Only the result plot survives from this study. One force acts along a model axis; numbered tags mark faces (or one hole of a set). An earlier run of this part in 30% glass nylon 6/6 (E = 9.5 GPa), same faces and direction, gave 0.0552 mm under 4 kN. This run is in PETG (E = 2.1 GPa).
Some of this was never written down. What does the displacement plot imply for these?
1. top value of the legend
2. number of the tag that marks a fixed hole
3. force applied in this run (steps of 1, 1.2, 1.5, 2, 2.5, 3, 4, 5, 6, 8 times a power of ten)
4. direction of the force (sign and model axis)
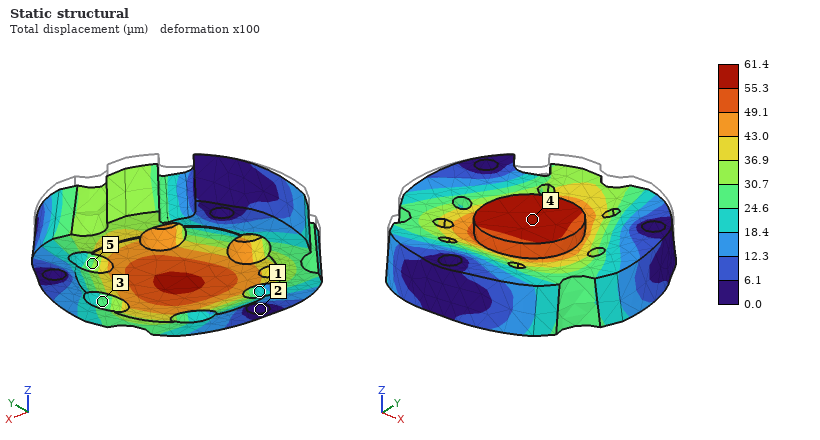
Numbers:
61.4 µm
2
1 kN
-Z
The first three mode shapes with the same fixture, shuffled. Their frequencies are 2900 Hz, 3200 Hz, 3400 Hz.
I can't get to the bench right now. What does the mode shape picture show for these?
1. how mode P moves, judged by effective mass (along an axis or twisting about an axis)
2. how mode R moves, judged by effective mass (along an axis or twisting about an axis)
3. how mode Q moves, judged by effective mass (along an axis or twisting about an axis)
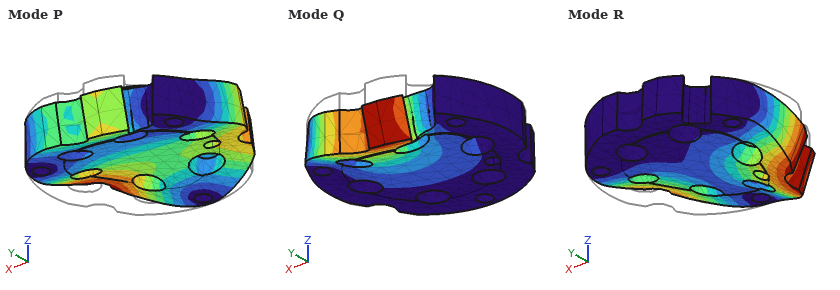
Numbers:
along Z
twisting about Y
along Z
